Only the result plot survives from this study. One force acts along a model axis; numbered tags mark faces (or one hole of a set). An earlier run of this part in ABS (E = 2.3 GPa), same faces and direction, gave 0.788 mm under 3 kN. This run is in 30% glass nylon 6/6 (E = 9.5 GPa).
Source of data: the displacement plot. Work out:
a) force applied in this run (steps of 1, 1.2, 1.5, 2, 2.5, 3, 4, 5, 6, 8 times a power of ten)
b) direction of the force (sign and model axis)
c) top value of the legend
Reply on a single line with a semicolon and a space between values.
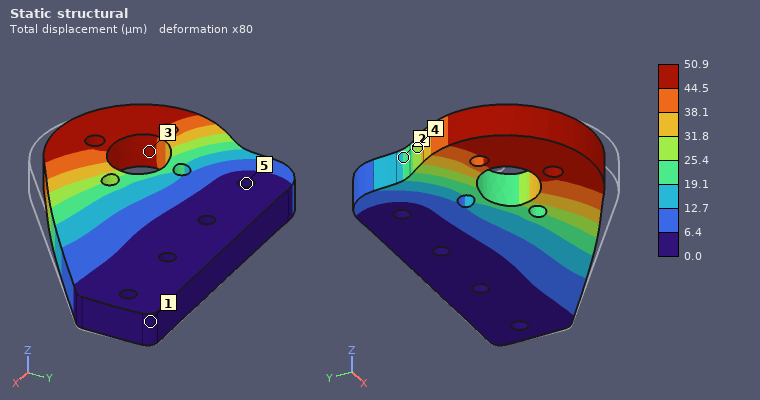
800 N; -X; 50.9 µm
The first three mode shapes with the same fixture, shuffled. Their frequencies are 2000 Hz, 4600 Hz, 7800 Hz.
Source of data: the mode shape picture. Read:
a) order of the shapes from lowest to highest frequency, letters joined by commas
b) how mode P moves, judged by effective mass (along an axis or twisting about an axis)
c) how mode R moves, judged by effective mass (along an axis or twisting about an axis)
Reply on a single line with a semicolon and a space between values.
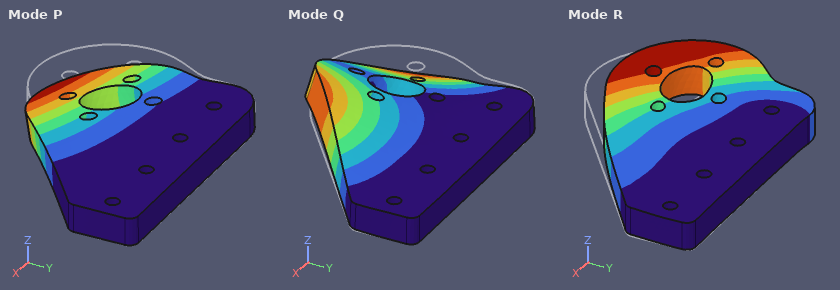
P, Q, R; along Z; along X
